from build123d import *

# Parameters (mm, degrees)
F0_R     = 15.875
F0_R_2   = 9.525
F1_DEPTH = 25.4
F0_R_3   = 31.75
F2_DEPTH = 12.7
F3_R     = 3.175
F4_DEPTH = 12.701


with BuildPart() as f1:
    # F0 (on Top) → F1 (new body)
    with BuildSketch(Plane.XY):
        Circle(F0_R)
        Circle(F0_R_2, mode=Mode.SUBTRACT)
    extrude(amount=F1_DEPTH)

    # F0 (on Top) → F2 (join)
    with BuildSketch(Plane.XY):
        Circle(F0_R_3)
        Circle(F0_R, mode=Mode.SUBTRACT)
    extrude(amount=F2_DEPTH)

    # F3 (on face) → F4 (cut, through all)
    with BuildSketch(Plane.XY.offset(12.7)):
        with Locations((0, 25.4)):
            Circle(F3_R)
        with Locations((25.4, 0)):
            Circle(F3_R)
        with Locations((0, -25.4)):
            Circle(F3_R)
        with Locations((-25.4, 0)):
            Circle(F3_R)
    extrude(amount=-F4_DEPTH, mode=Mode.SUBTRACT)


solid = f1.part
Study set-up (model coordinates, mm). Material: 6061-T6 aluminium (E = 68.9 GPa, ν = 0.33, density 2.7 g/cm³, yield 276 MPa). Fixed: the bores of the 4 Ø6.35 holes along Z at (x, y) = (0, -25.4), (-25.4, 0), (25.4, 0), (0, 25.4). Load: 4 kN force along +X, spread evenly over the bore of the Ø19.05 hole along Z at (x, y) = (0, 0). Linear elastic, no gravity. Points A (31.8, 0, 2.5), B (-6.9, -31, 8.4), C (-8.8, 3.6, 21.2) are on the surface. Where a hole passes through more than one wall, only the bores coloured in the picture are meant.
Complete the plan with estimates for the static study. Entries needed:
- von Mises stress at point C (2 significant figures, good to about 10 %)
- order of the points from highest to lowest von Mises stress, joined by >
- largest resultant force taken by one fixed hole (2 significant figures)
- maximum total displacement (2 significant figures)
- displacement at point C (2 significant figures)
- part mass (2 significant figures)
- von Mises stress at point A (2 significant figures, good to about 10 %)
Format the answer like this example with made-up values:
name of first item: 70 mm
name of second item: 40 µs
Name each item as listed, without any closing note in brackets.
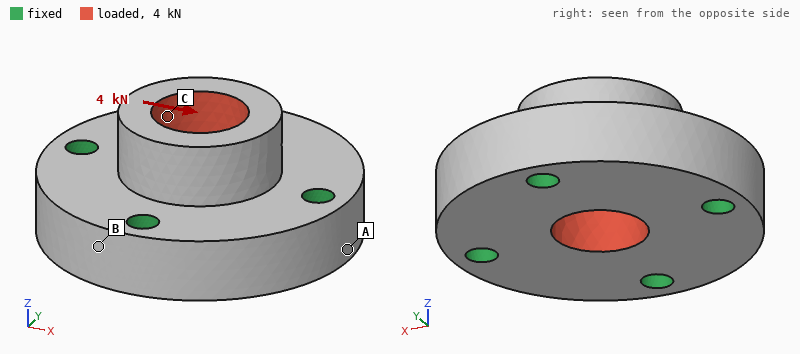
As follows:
von Mises stress at point C: 5.6 MPa
order of the points from highest to lowest von Mises stress, joined by >: C > A > B
largest resultant force taken by one fixed hole: 1.3 kN
maximum total displacement: 5.0 µm
displacement at point C: 3.9 µm
part mass: 110 g
von Mises stress at point A: 3.2 MPa
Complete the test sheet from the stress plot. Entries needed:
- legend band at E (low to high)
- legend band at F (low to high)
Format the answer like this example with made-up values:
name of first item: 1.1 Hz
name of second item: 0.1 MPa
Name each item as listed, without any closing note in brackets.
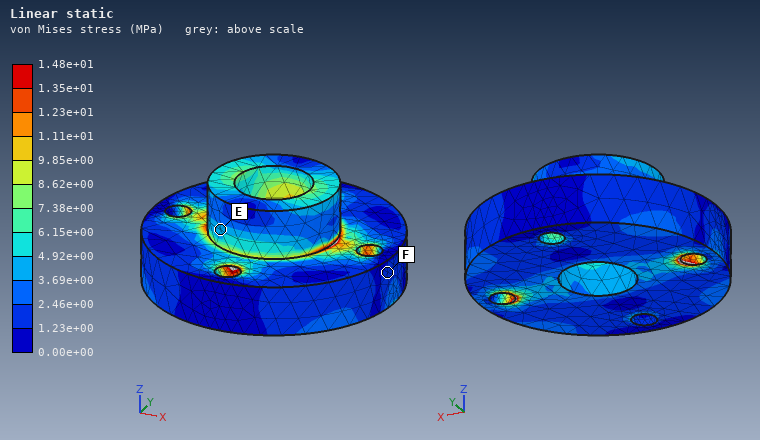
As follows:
legend band at E: 3.69e+00 to 4.92e+00 MPa
legend band at F: 1.23e+00 to 2.46e+00 MPa
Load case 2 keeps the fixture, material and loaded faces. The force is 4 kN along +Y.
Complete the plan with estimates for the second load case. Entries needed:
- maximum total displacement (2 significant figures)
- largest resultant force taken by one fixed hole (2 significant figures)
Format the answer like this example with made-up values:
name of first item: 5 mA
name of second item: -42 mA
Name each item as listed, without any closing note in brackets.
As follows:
maximum total displacement: 5.0 µm
largest resultant force taken by one fixed hole: 1.3 kN
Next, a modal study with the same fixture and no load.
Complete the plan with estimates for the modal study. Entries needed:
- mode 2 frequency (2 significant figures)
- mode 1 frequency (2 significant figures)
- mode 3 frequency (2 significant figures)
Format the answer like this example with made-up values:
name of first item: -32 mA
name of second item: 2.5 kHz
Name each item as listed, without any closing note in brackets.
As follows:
mode 2 frequency: 26 kHz
mode 1 frequency: 26 kHz
mode 3 frequency: 26 kHz
